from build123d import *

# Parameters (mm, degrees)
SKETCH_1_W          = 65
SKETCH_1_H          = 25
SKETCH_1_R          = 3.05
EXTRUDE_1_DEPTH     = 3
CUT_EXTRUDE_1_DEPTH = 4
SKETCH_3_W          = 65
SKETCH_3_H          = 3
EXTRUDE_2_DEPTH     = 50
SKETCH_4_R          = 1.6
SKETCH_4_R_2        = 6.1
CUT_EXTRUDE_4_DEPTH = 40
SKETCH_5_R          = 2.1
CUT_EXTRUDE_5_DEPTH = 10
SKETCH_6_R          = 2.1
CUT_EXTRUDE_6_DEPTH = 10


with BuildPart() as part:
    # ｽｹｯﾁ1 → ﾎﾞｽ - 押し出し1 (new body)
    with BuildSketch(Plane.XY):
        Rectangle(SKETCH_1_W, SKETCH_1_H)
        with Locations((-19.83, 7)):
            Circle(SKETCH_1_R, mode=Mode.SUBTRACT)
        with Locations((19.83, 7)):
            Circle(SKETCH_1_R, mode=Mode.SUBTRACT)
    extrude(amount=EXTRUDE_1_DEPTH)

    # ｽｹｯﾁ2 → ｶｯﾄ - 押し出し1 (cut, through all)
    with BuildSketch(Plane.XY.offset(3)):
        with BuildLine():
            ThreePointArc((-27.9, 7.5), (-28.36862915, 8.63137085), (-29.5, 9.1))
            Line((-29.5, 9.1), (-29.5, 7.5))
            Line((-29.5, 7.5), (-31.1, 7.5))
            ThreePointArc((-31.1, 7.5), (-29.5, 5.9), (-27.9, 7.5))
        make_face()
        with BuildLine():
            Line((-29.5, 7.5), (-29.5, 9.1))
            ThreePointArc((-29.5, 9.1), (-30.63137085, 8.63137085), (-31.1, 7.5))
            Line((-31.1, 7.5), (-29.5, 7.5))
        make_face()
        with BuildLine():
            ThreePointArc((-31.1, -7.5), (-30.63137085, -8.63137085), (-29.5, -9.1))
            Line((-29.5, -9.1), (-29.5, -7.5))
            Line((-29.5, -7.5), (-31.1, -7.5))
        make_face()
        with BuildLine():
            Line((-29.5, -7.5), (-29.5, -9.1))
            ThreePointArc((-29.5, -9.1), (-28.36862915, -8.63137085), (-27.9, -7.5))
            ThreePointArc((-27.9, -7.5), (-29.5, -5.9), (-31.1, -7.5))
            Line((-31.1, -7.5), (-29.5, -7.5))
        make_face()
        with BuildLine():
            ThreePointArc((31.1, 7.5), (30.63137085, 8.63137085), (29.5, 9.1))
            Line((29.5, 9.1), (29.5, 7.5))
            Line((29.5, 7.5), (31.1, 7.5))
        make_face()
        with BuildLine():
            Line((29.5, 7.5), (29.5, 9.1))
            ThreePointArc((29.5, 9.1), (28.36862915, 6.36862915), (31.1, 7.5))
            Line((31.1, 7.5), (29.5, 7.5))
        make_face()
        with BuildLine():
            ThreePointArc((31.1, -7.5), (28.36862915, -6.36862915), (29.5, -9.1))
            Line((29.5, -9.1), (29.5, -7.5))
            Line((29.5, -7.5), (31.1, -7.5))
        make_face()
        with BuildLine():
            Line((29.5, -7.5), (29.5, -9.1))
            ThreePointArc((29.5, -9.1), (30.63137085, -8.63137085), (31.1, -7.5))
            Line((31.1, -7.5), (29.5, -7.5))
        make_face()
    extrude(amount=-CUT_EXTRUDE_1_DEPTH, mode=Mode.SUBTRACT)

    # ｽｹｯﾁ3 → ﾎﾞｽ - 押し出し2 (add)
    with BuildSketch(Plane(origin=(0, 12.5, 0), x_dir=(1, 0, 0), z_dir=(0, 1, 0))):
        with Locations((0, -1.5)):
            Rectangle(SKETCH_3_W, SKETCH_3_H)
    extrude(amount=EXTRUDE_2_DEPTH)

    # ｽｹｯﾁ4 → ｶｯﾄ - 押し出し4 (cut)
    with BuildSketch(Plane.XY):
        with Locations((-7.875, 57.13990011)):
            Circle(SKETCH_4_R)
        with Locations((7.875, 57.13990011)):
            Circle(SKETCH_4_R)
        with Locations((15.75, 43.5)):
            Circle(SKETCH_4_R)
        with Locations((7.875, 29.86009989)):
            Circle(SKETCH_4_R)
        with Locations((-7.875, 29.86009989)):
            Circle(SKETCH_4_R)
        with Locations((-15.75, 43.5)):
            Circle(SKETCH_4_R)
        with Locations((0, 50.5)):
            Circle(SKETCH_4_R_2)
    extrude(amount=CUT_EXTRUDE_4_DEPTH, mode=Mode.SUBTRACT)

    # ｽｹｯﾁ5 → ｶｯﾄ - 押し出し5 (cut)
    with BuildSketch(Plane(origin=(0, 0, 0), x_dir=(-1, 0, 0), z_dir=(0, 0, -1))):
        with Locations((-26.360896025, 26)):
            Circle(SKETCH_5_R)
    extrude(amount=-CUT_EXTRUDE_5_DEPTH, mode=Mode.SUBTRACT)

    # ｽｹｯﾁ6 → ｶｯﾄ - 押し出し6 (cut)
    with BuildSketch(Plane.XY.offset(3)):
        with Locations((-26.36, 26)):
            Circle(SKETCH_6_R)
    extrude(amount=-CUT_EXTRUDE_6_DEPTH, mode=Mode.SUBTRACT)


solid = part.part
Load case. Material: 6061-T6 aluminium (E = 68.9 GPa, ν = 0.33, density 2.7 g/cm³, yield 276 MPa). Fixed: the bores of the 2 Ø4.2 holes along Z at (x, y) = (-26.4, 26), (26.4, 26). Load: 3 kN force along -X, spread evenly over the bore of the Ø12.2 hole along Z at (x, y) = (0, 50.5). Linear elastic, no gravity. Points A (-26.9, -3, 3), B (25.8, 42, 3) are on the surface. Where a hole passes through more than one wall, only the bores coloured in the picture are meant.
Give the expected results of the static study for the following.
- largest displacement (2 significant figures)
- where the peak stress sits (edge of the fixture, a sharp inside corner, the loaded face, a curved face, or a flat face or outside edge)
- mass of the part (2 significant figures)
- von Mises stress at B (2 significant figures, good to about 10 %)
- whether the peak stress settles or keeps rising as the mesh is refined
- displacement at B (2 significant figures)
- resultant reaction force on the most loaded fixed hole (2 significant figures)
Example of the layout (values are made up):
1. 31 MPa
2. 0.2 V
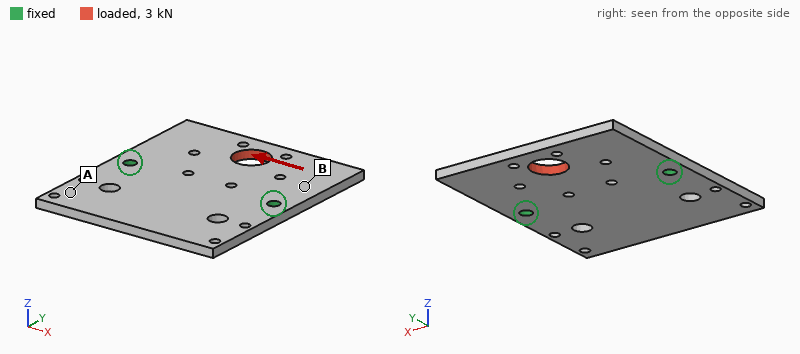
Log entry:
1. 37 µm
2. edge of the fixture
3. 37 g
4. 21 MPa
5. keeps rising
6. 17 µm
7. 2.0 kN
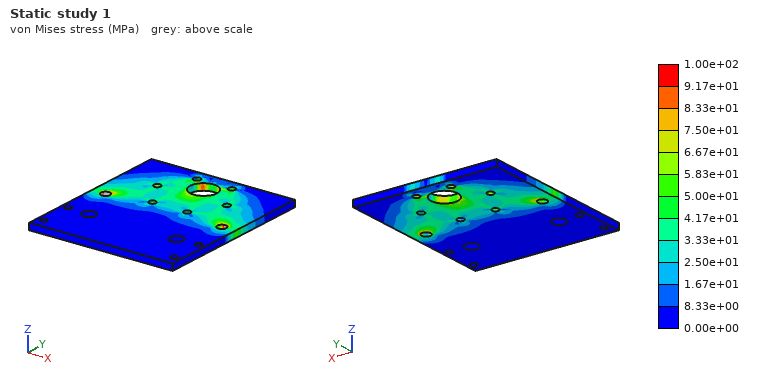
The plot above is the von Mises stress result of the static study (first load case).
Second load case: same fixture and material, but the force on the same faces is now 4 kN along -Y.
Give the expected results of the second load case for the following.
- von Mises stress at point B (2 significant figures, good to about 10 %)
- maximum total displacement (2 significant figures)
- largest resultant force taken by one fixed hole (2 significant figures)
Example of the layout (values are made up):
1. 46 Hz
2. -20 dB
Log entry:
1. 18 MPa
2. 35 µm
3. 2.1 kN
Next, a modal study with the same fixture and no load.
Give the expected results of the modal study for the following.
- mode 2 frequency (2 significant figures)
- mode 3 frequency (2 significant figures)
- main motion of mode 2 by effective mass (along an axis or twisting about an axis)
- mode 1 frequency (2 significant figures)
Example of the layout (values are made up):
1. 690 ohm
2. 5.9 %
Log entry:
1. 1800 Hz
2. 2800 Hz
3. along Z
4. 1300 Hz
